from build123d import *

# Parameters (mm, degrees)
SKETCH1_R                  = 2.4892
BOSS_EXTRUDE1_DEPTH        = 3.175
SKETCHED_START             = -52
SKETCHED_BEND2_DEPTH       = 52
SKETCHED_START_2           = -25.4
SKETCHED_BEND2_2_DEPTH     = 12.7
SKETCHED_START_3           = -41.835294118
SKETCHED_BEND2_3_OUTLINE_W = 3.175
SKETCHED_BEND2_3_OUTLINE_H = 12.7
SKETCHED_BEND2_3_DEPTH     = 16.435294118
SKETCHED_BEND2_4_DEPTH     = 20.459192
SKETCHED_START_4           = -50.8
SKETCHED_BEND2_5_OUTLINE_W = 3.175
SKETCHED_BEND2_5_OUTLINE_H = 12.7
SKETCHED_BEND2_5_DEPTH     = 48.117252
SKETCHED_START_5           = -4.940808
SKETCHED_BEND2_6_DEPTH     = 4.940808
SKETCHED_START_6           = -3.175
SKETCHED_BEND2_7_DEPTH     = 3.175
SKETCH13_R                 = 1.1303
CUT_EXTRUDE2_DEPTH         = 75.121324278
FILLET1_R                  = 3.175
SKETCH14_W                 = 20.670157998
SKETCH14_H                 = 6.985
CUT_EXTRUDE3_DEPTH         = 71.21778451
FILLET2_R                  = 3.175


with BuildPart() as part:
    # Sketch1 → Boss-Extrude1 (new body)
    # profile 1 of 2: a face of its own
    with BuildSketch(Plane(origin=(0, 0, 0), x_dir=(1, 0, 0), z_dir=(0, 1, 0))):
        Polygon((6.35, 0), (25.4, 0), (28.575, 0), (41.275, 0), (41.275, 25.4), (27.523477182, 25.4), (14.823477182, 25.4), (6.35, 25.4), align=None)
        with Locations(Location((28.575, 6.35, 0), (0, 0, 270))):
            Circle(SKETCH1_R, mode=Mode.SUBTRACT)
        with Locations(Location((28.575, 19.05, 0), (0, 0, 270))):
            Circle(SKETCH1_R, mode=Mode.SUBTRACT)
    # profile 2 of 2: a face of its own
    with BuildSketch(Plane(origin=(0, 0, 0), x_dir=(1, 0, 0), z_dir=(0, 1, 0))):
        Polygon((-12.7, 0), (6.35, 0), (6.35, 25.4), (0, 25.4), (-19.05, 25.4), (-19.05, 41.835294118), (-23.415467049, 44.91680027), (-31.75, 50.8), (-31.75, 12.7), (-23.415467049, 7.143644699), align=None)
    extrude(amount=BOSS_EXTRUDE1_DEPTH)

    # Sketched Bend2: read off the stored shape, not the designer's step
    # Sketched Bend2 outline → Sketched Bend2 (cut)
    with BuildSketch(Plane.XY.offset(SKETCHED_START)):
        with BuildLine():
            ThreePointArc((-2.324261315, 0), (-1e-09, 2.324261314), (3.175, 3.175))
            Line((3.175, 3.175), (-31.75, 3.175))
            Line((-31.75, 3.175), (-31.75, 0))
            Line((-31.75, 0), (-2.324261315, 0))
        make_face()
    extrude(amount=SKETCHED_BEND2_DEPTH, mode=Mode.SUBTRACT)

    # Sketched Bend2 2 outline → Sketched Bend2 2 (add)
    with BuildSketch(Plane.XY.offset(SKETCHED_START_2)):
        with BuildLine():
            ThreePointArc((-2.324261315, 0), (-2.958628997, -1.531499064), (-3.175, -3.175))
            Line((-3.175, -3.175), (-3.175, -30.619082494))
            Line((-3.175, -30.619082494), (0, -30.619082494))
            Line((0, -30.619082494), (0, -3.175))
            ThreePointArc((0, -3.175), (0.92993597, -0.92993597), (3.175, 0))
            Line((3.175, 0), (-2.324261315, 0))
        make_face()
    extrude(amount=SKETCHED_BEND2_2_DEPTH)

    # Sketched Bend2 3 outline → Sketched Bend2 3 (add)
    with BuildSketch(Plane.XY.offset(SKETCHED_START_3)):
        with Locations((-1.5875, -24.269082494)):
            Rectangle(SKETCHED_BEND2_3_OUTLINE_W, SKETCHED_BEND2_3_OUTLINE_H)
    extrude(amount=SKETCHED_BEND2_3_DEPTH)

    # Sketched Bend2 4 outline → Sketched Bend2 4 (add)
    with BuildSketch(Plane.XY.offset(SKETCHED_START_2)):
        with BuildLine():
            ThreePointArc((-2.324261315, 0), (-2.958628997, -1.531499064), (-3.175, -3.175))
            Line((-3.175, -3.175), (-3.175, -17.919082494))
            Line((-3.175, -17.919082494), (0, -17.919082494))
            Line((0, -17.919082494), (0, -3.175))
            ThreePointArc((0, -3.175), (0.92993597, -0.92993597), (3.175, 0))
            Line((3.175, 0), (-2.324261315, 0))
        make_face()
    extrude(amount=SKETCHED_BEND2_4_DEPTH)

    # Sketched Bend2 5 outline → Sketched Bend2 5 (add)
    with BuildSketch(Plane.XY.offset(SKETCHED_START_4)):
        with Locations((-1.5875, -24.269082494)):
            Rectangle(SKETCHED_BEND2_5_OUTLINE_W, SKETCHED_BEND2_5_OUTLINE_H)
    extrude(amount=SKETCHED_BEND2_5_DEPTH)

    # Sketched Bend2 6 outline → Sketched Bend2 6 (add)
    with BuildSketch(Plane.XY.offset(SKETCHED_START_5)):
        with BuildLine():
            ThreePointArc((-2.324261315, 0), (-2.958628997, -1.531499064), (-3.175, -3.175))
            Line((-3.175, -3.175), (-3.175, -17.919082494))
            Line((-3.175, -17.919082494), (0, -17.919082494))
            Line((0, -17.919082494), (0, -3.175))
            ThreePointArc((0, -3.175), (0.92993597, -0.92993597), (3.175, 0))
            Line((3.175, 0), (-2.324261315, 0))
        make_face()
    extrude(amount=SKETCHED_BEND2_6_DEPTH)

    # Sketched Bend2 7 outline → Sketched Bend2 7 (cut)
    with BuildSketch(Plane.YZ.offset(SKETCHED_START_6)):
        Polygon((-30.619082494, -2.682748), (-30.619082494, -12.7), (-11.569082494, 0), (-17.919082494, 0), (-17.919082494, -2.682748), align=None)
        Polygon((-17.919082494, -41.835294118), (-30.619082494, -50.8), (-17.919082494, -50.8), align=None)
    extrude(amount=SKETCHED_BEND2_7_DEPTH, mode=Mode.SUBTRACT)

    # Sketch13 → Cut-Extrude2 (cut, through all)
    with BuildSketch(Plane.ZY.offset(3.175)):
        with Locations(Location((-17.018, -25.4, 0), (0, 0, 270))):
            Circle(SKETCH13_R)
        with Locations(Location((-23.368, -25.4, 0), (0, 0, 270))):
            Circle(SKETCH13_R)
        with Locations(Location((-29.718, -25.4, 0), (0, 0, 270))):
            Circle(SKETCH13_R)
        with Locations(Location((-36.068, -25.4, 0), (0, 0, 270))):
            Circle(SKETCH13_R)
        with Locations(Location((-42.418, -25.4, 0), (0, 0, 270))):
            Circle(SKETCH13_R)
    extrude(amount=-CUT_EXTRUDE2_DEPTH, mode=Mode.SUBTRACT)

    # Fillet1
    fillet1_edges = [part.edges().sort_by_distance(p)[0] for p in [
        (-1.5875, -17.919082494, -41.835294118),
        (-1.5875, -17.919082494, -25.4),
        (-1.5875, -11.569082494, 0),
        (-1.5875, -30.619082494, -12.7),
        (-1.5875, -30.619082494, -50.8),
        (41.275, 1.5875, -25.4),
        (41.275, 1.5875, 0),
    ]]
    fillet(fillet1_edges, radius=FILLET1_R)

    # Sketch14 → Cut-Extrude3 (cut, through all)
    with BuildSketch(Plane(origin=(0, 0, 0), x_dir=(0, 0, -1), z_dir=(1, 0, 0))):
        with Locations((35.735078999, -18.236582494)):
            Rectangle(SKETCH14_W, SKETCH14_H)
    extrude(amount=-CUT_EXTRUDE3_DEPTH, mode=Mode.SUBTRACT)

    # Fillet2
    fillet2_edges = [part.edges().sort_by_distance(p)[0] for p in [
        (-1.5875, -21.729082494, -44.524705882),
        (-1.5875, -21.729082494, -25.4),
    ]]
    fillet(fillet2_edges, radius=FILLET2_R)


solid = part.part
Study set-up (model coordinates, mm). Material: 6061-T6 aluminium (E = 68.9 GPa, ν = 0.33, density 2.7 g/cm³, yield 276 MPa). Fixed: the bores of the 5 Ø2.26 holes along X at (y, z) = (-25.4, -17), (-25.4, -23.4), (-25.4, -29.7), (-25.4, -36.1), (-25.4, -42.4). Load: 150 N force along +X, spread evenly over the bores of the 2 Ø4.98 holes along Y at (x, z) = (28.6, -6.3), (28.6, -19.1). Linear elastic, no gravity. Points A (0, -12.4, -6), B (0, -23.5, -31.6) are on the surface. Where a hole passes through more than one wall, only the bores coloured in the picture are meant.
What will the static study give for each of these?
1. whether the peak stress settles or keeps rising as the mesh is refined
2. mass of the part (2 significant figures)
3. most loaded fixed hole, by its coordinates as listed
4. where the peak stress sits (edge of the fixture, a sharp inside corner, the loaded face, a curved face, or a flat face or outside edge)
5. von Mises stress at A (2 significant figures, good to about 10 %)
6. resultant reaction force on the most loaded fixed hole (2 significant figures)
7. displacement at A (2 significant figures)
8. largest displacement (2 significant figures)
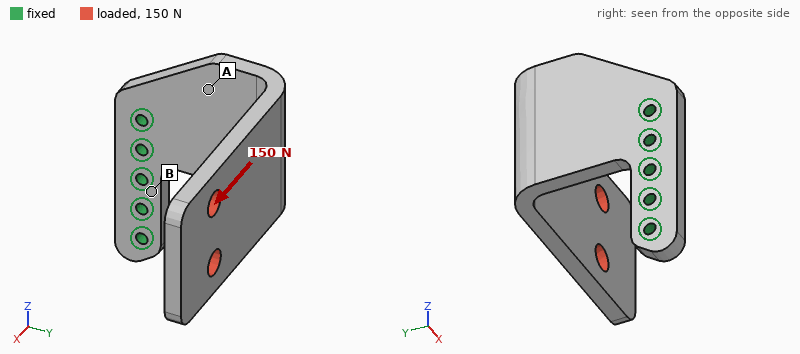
keeps rising
16 g
(-25.4, -17)
edge of the fixture
40 MPa
160 N
0.12 mm
0.74 mm
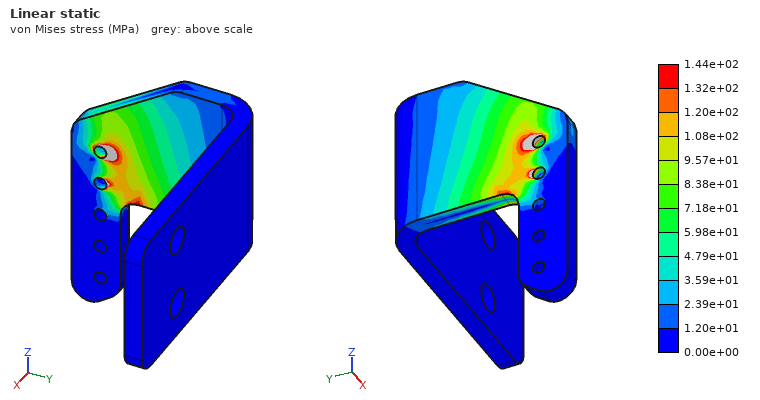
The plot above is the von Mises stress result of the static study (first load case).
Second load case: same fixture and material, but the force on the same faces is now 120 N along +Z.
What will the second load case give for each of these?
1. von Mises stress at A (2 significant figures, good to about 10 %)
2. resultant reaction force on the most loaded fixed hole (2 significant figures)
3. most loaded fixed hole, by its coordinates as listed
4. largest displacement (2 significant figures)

55 MPa
450 N
(-25.4, -17)
0.70 mm
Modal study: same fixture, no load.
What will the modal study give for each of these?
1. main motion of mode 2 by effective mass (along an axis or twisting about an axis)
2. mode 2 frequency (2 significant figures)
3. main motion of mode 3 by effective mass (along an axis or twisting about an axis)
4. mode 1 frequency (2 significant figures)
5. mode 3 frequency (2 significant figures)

along Z
1000 Hz
along X
660 Hz
2100 Hz
